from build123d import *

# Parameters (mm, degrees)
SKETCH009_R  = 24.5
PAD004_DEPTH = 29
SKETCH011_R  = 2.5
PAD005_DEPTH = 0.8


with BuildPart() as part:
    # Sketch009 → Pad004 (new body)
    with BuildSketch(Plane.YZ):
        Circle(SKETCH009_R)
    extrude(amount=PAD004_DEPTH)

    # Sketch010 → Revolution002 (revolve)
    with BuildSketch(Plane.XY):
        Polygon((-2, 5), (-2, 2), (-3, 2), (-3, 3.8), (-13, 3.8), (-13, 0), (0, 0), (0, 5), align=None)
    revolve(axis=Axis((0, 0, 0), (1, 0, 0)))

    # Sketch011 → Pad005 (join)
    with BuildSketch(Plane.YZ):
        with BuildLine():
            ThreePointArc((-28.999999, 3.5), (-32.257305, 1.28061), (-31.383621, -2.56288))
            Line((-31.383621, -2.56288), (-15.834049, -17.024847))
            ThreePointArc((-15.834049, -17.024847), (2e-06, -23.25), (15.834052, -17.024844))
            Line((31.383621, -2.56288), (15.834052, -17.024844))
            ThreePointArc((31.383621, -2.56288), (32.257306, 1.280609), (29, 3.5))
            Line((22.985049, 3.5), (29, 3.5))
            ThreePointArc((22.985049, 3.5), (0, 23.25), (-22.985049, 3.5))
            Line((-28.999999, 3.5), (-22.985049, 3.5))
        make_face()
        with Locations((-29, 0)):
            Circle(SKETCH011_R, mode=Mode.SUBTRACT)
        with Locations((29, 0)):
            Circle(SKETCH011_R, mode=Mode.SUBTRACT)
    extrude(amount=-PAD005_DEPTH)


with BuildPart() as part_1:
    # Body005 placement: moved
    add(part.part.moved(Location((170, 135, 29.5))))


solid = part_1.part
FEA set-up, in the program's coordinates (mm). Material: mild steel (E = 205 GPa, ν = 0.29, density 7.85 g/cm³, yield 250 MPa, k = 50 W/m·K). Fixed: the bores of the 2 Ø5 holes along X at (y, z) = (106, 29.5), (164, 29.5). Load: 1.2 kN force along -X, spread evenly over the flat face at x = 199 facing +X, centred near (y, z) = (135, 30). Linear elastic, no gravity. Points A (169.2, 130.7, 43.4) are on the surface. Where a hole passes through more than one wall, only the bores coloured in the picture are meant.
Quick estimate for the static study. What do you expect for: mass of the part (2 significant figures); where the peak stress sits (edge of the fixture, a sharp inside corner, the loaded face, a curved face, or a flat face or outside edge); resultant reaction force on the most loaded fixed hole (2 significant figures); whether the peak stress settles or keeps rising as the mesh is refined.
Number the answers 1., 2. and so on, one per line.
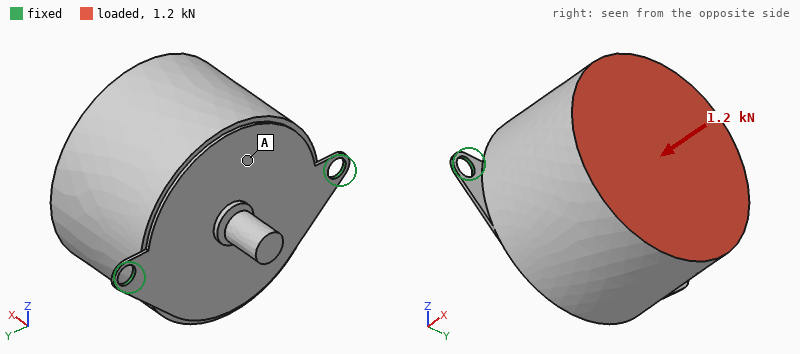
1. 450 g
2. edge of the fixture
3. 710 N
4. keeps rising
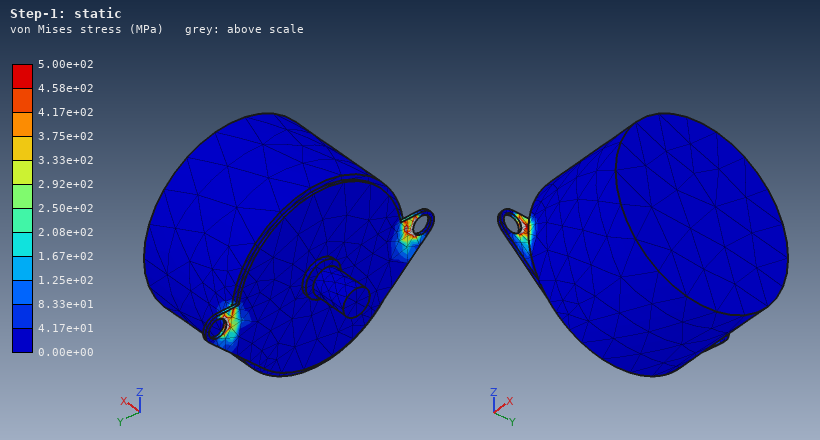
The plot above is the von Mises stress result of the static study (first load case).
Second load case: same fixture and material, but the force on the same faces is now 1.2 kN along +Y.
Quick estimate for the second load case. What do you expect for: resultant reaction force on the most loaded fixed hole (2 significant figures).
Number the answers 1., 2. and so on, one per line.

1. 920 N
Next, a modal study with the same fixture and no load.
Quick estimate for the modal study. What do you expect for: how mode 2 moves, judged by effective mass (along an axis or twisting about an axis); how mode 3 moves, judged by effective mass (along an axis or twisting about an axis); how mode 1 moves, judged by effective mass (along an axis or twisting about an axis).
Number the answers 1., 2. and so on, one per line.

1. along X
2. along Y
3. along Z
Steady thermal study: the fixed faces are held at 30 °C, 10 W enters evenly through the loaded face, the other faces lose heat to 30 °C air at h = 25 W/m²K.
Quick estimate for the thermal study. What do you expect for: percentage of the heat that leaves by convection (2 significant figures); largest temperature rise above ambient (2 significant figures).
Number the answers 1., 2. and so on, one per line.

1. 50 %
2. 31 K
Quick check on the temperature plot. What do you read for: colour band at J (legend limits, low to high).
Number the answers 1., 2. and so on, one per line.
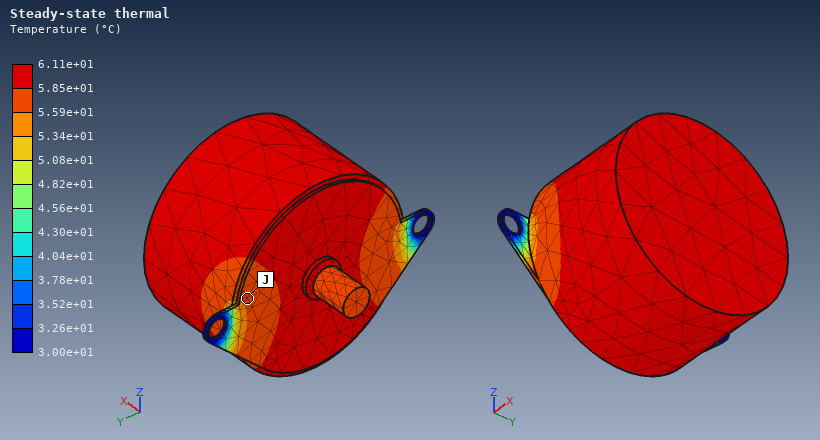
1. 5.59e+01 to 5.85e+01 °C
